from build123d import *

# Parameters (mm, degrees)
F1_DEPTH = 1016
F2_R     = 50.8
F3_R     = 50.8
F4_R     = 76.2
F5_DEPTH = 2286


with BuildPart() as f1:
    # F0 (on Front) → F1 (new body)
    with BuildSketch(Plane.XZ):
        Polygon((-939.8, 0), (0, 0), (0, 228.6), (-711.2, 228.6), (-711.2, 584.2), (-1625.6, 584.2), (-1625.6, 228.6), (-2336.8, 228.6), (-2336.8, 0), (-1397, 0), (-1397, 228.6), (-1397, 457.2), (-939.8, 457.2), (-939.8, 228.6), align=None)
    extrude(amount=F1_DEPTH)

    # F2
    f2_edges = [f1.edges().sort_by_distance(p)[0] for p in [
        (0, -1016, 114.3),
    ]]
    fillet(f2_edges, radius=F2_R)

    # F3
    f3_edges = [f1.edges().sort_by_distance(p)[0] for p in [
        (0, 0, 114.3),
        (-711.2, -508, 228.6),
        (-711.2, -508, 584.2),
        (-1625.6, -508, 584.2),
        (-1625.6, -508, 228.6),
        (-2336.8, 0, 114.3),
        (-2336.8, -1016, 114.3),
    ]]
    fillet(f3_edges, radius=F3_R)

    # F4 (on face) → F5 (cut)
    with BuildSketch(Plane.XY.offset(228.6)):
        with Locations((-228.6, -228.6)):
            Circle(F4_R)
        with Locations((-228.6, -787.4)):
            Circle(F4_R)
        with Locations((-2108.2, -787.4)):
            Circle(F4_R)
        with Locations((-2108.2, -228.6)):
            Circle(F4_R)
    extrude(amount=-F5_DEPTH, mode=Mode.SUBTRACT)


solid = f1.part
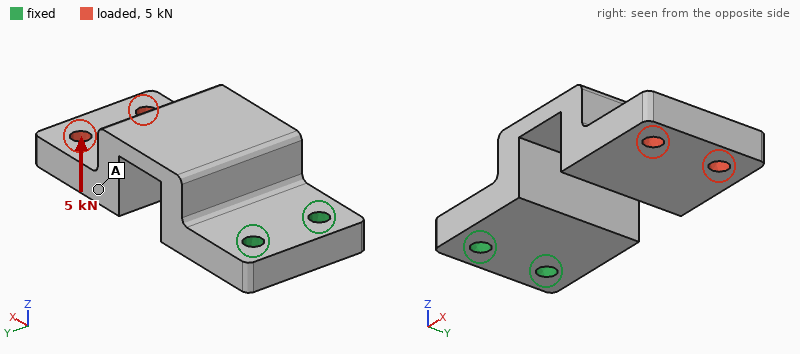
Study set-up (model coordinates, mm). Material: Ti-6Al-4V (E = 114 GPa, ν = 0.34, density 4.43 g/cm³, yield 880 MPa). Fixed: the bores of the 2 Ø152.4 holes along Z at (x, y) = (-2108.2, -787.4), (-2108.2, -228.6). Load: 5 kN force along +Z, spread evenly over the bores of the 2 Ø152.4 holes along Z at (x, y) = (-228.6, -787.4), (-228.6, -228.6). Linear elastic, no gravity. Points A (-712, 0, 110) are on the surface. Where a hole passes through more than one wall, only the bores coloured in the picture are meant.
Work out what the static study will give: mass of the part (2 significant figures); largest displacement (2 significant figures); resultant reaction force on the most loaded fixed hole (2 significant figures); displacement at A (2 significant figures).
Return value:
2900 kg
0.27 mm
2.6 kN
0.13 mm
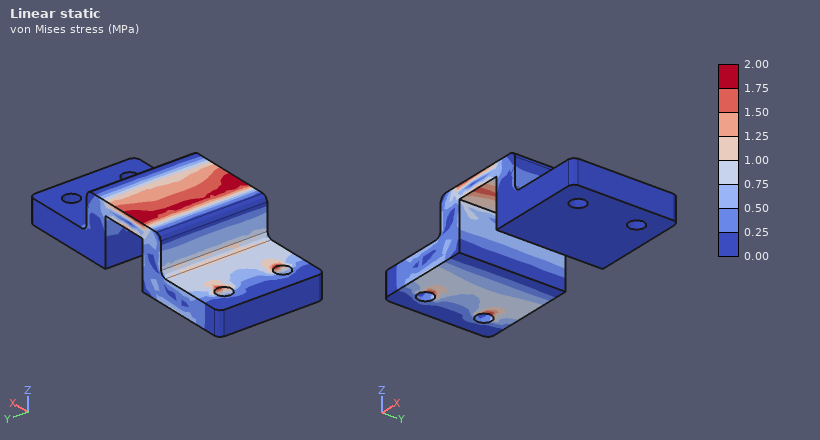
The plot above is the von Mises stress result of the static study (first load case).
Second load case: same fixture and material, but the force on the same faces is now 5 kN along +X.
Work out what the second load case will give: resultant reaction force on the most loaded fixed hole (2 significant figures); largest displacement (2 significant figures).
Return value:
2.5 kN
76 µm
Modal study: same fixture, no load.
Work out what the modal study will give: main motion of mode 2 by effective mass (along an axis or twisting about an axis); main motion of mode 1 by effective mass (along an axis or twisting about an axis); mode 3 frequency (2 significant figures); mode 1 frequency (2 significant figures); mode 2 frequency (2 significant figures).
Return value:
along Y
along Z
91 Hz
28 Hz
65 Hz
